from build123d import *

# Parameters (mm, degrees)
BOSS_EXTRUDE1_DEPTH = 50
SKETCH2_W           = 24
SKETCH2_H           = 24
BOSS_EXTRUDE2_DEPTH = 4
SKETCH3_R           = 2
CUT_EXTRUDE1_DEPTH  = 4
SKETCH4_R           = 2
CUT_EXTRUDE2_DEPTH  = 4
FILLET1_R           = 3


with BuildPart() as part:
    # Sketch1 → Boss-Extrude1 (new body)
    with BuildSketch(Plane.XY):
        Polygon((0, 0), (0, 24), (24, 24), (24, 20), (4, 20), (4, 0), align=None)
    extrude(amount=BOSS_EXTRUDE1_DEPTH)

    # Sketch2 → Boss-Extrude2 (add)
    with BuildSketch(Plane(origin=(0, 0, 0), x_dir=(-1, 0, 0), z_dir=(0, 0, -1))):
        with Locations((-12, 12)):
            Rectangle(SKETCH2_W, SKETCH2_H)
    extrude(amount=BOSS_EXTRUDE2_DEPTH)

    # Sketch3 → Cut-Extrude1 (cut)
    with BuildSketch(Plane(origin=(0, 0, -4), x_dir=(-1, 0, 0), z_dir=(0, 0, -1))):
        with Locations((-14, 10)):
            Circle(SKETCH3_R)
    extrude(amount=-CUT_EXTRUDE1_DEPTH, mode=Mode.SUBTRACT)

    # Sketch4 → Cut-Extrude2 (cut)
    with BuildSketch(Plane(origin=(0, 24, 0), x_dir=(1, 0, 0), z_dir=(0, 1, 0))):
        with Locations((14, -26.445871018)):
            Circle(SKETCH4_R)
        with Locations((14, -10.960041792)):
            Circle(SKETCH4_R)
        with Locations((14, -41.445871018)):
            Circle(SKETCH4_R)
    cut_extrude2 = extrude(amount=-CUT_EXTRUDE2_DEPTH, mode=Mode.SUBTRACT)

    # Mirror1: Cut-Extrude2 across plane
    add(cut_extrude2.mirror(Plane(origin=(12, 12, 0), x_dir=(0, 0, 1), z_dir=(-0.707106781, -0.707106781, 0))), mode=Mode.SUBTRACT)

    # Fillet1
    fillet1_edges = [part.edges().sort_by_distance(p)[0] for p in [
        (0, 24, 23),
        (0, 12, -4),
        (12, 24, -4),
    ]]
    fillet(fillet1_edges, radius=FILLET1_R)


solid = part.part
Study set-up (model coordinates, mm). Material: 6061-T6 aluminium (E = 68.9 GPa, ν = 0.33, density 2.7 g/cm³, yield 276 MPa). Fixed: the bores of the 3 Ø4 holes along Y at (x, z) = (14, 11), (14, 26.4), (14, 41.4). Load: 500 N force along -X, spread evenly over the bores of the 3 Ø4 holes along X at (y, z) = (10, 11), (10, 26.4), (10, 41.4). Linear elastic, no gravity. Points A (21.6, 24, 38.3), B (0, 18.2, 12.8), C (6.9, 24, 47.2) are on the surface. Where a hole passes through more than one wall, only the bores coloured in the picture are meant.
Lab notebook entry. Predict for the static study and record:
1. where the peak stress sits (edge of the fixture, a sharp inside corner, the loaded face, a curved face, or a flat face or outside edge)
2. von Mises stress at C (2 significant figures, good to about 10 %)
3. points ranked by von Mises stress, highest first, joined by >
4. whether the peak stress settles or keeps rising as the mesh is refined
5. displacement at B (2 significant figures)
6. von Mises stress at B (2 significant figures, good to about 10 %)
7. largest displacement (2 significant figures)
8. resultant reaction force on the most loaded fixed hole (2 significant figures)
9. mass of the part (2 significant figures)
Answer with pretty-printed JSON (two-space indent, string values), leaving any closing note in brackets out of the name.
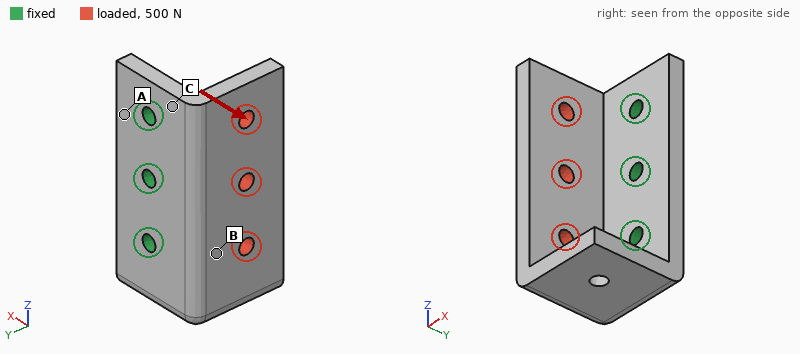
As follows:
{
  "where the peak stress sits": "edge of the fixture",
  "von Mises stress at C": "34 MPa",
  "points ranked by von Mises stress, highest first, joined by >": "C > B > A",
  "whether the peak stress settles or keeps rising as the mesh is refined": "keeps rising",
  "displacement at B": "26 µm",
  "von Mises stress at B": "18 MPa",
  "largest displacement": "96 µm",
  "resultant reaction force on the most loaded fixed hole": "180 N",
  "mass of the part": "29 g"
}
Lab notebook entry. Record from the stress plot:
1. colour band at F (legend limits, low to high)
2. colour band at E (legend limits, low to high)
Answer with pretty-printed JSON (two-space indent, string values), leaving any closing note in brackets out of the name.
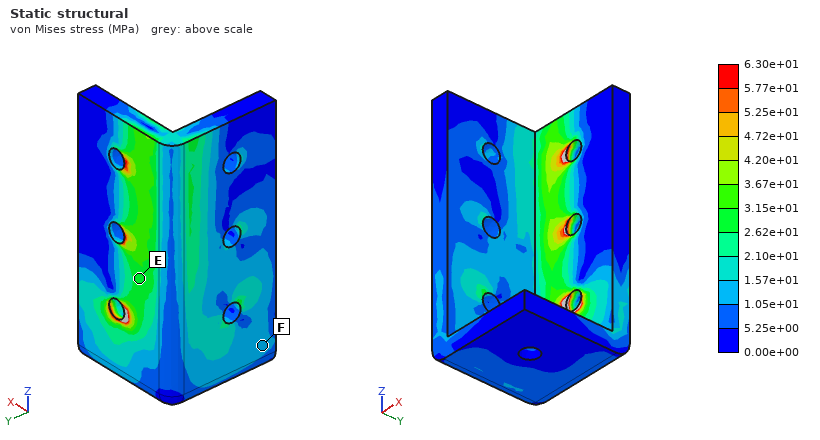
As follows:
{
  "colour band at F": "1.05e+01 to 1.57e+01 MPa",
  "colour band at E": "2.62e+01 to 3.15e+01 MPa"
}
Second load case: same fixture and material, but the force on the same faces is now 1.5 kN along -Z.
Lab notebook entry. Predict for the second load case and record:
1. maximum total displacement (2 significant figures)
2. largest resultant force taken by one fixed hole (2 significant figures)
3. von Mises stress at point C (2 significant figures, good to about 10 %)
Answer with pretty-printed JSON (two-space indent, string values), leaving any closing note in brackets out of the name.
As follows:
{
  "maximum total displacement": "72 µm",
  "largest resultant force taken by one fixed hole": "900 N",
  "von Mises stress at point C": "19 MPa"
}
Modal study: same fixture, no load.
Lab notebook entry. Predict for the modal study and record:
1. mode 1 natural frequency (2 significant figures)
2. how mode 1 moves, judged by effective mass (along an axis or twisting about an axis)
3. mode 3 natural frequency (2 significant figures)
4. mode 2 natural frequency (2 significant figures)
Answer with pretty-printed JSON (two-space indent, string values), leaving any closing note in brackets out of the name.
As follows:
{
  "mode 1 natural frequency": "3900 Hz",
  "how mode 1 moves, judged by effective mass": "along X",
  "mode 3 natural frequency": "7600 Hz",
  "mode 2 natural frequency": "5100 Hz"
}
